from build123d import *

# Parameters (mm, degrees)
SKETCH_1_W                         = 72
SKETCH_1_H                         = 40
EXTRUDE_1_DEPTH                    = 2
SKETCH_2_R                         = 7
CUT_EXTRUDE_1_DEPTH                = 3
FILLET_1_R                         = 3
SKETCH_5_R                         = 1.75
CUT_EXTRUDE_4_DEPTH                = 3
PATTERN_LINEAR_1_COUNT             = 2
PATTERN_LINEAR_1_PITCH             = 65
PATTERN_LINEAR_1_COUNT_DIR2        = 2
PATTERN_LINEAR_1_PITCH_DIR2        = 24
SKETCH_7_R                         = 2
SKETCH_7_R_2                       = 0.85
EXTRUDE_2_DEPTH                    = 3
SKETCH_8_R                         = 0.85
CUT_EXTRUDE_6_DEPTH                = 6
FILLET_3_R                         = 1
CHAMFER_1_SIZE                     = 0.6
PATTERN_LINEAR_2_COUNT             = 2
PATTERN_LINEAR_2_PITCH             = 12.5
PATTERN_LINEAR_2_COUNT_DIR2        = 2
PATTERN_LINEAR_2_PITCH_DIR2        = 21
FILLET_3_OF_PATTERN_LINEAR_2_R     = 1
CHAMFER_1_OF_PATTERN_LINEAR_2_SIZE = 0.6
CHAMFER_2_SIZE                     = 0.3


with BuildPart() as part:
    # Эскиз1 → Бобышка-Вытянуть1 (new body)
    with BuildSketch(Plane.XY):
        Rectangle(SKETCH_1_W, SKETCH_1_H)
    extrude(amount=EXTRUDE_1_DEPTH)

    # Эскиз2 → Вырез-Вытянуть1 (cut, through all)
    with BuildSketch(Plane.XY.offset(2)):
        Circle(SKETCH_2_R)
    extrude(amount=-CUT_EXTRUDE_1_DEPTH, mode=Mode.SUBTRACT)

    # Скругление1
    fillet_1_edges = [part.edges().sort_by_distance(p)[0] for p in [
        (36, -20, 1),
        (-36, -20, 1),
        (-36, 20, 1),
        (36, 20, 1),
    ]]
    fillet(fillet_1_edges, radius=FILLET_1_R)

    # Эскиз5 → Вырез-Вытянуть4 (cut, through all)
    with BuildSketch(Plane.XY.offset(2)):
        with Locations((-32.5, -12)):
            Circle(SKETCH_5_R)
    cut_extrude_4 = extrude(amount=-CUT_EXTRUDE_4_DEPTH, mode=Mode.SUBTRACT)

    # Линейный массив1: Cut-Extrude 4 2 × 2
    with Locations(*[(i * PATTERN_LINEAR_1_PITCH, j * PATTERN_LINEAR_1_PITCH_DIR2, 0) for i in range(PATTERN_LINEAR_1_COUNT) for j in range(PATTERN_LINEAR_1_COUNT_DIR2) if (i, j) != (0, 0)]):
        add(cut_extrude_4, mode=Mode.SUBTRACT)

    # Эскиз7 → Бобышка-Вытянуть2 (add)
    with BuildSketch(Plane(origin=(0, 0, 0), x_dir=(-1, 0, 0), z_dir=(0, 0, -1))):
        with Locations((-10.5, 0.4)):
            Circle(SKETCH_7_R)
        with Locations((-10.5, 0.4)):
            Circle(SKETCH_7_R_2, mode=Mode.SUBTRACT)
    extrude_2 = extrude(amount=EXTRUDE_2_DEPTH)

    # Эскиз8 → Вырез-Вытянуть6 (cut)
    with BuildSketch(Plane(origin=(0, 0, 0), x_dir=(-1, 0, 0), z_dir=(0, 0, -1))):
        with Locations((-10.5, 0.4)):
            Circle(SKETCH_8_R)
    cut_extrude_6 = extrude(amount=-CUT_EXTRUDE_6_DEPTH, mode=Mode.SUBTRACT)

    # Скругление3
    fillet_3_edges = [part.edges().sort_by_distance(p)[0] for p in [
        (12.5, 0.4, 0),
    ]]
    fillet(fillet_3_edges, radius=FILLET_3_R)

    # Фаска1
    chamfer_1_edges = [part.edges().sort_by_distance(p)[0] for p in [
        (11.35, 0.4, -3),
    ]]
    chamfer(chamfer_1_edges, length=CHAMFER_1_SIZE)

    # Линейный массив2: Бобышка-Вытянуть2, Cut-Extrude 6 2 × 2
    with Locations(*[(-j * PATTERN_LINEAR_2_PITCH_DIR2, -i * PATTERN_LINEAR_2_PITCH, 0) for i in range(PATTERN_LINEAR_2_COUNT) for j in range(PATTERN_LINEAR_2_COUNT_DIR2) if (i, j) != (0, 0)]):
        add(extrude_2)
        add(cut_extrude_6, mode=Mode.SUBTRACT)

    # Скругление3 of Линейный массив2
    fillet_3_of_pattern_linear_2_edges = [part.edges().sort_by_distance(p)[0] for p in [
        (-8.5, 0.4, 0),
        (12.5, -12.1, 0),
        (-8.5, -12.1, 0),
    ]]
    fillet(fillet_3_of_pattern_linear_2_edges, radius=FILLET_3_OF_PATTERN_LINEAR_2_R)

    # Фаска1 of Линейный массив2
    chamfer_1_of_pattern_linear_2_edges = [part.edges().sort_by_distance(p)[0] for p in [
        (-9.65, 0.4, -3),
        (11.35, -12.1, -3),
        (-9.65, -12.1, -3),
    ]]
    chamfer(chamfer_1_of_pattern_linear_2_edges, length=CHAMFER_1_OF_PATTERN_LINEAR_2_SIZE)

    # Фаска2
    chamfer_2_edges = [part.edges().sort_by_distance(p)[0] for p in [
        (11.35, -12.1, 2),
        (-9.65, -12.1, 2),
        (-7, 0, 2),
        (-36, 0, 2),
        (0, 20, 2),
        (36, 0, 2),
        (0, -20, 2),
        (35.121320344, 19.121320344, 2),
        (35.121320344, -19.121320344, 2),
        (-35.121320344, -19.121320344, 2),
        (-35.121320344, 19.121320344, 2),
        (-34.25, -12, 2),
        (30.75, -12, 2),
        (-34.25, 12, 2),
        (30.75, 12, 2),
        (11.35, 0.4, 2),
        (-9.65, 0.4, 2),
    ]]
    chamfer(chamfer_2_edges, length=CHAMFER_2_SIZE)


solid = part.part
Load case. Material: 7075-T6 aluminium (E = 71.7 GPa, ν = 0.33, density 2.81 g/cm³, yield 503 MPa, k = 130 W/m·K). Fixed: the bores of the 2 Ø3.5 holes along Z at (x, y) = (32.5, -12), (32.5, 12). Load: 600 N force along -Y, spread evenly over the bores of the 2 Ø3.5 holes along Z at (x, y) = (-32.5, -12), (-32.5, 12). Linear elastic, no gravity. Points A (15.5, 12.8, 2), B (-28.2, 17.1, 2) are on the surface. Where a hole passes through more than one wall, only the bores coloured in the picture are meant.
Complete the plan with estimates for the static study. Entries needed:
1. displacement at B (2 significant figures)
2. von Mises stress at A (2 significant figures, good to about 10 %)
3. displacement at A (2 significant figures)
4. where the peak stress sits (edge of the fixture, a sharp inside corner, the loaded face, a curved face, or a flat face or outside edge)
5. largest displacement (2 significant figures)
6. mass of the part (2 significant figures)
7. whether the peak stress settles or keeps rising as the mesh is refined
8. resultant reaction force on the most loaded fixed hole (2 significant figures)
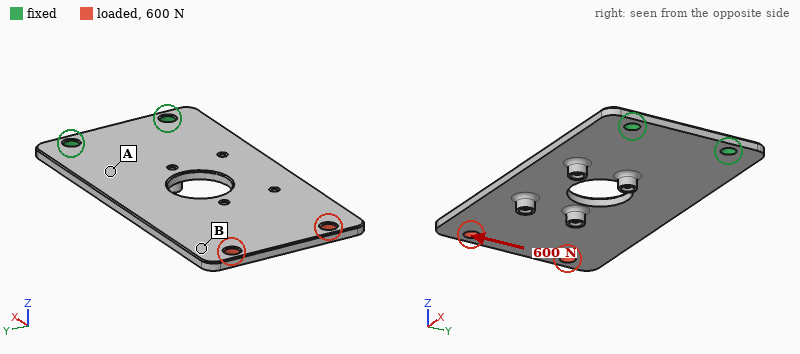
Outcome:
0.12 mm
35 MPa
0.024 mm
edge of the fixture
0.15 mm
15 g
keeps rising
1.5 kN
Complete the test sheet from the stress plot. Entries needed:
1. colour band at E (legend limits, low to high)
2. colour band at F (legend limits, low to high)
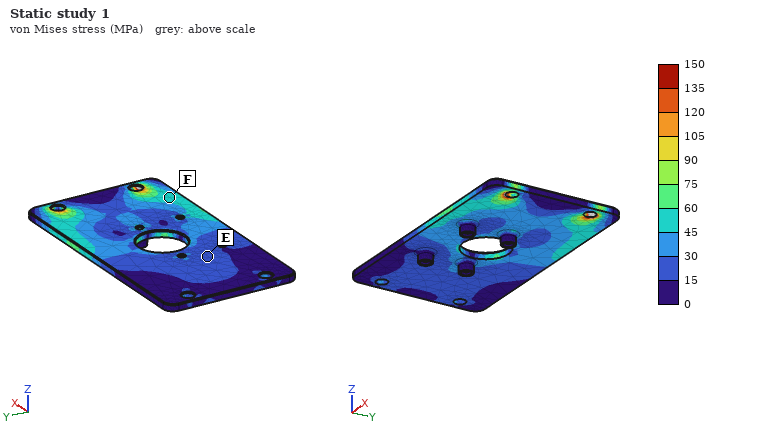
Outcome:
15 to 30 MPa
45 to 60 MPa
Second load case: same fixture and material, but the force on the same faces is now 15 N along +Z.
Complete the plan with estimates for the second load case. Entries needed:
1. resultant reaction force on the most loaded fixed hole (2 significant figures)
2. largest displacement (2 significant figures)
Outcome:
7.6 N
0.84 mm
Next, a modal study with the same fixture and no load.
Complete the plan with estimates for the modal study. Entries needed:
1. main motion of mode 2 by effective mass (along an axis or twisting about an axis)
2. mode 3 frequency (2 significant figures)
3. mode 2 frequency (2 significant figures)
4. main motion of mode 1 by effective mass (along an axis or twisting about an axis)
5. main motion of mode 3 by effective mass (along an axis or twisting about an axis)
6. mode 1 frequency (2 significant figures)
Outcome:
twisting about X
2100 Hz
1300 Hz
along Z
along Z
340 Hz
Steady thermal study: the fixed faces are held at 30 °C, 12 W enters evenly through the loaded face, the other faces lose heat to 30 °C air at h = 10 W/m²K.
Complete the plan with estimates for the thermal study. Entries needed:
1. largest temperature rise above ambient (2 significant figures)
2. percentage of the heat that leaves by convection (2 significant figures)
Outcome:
82 K
19 %
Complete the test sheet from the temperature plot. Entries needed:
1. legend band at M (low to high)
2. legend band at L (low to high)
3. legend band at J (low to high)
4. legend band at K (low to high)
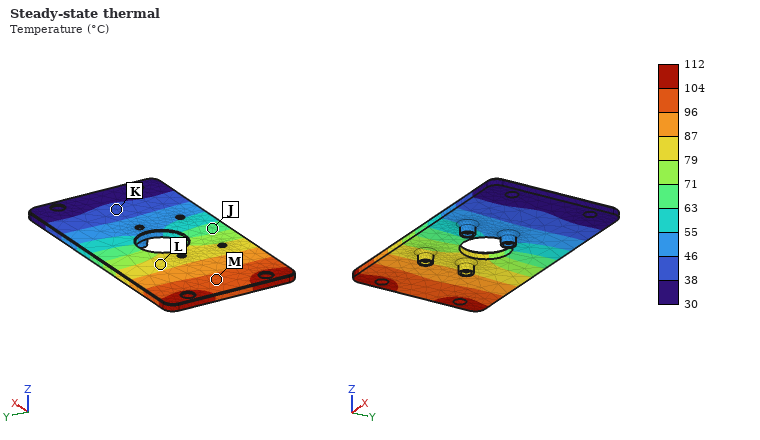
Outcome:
96 to 104 °C
79 to 87 °C
63 to 71 °C
38 to 46 °C
